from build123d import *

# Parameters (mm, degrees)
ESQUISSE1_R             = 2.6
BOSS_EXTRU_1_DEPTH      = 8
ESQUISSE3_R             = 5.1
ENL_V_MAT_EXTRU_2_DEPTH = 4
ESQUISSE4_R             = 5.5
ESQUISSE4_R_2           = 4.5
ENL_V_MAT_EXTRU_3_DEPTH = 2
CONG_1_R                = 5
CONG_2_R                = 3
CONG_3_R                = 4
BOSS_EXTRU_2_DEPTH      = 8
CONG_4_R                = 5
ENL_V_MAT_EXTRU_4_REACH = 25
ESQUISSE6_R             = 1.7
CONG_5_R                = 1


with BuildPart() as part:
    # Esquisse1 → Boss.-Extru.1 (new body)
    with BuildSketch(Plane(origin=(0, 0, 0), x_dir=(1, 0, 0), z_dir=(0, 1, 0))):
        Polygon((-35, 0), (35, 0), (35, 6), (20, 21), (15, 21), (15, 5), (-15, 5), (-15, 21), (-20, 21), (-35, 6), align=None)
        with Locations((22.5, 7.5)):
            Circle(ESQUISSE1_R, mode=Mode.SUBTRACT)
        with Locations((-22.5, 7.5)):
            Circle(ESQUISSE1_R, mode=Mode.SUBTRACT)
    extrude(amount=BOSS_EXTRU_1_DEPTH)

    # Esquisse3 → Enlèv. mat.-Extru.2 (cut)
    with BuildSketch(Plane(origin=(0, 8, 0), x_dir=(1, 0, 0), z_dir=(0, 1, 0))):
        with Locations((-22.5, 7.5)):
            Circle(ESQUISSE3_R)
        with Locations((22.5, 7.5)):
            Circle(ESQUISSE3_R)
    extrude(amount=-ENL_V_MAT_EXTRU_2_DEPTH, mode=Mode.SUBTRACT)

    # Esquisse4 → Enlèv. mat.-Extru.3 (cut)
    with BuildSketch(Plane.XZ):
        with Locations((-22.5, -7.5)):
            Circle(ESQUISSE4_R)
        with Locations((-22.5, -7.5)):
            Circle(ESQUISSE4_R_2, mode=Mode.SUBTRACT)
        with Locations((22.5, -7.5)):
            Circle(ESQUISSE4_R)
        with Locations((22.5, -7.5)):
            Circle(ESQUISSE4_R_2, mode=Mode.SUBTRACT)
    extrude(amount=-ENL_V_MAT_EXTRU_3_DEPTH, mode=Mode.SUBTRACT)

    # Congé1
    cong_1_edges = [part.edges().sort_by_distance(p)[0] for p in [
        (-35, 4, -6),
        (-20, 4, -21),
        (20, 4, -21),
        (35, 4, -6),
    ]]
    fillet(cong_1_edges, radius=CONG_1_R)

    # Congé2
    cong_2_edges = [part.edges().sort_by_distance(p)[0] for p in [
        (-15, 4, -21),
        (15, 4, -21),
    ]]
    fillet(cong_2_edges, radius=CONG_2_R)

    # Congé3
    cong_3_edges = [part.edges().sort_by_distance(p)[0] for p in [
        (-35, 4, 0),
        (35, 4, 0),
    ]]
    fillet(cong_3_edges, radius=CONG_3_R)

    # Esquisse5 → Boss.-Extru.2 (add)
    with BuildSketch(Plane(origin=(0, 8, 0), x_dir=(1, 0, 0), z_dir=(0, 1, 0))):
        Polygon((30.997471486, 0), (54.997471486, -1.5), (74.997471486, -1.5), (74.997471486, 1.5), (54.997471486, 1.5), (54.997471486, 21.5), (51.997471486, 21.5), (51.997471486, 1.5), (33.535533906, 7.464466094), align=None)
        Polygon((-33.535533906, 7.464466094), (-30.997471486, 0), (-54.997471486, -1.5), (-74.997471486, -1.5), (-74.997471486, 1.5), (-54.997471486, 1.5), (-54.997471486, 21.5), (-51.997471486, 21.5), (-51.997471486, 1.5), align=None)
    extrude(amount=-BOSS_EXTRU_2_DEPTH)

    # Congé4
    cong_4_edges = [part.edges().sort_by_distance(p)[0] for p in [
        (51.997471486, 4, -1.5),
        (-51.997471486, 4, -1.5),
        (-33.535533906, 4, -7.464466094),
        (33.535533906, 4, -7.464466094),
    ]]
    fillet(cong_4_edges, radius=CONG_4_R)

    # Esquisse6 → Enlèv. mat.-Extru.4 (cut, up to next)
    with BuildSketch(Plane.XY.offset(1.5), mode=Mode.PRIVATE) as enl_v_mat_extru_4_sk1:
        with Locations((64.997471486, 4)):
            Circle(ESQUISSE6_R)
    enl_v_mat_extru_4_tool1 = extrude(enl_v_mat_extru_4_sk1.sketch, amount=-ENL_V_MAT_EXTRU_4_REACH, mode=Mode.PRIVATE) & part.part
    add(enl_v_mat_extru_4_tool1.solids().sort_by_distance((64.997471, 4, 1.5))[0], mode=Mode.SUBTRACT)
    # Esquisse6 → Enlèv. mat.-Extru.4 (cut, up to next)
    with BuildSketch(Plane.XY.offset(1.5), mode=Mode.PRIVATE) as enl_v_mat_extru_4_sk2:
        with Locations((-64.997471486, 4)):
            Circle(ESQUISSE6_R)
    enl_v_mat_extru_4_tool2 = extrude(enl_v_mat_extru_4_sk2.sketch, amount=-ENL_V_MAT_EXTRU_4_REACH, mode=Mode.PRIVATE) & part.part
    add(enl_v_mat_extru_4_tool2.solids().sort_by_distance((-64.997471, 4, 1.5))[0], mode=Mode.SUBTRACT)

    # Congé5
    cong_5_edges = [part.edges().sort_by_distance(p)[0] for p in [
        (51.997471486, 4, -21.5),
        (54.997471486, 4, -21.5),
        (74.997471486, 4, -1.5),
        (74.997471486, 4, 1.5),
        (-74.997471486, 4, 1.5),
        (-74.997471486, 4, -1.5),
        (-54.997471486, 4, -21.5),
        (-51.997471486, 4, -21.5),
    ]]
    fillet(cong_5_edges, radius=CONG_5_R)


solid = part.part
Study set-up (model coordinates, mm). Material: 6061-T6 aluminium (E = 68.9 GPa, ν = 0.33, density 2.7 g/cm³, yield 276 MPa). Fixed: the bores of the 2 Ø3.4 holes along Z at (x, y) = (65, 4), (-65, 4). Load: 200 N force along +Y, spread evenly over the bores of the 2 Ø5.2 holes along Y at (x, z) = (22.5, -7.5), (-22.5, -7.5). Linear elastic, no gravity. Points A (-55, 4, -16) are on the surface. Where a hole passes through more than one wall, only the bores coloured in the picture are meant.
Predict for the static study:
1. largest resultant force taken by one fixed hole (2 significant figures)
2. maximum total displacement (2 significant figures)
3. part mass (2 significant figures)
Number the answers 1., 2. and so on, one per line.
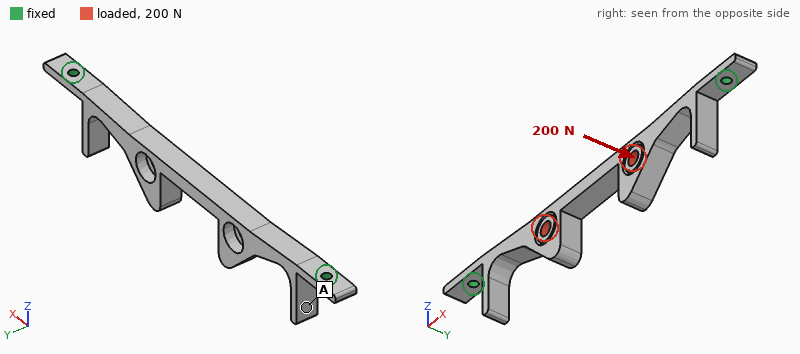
1. 100 N
2. 0.28 mm
3. 23 g
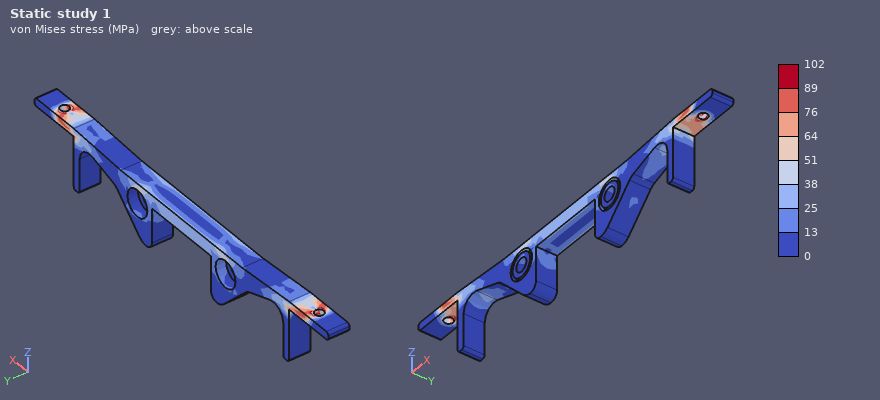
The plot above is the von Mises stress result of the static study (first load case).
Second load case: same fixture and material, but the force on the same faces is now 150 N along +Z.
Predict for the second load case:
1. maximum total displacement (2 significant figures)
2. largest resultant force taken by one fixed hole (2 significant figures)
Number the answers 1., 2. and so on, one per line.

1. 0.22 mm
2. 400 N
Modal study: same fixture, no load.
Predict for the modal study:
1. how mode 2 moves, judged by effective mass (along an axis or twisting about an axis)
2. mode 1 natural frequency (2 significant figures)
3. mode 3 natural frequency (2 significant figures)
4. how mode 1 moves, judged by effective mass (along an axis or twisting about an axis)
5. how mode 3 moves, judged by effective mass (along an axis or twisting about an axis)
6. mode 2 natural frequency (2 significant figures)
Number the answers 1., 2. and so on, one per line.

1. along Y
2. 1200 Hz
3. 3000 Hz
4. along Z
5. twisting about X
6. 1300 Hz
